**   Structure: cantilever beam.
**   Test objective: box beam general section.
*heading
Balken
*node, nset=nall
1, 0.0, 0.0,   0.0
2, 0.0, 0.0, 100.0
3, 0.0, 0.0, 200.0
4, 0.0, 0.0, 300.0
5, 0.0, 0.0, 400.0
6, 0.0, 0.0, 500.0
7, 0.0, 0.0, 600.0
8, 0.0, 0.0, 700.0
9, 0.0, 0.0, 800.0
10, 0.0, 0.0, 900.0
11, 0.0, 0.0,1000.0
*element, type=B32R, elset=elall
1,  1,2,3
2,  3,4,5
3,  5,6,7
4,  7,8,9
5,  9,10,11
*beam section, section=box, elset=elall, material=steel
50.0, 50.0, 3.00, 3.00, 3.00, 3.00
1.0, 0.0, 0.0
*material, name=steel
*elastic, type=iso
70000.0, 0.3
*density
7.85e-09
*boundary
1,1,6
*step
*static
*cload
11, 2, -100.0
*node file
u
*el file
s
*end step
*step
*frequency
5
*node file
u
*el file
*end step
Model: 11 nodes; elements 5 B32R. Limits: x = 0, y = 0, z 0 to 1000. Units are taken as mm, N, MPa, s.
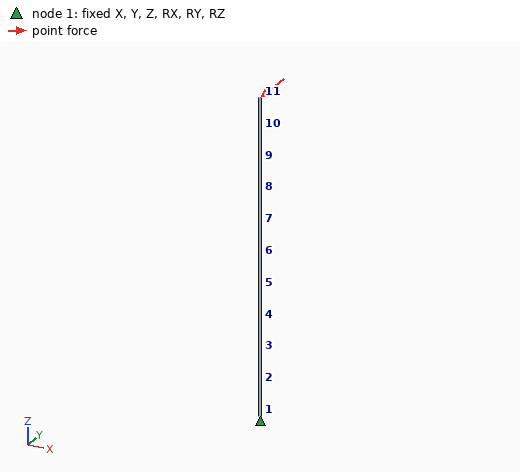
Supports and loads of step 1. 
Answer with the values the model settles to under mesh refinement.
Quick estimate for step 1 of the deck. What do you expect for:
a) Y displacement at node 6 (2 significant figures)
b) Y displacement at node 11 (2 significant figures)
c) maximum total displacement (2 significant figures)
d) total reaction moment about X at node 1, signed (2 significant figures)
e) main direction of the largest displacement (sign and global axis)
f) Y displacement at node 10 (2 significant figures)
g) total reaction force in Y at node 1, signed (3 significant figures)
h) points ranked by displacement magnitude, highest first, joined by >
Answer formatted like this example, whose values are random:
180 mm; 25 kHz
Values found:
-0.72 mm; -2.3 mm; 2.3 mm; -100000 N·mm; -Y; -2.0 mm; 100 N; node 11 > node 10 > node 8 > node 6 > node 1
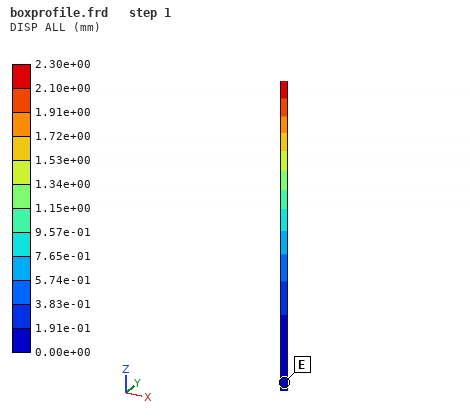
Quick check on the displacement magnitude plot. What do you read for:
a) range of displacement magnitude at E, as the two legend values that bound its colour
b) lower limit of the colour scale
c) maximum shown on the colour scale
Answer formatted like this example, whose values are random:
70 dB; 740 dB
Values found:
0.00e+00 to 1.91e-01 mm; 0.00e+00 mm; 2.30e+00 mm
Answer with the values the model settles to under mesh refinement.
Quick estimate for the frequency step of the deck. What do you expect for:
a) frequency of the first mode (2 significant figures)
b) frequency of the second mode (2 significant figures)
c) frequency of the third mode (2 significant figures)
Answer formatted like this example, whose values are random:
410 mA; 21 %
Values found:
32 Hz; 32 Hz; 190 Hz
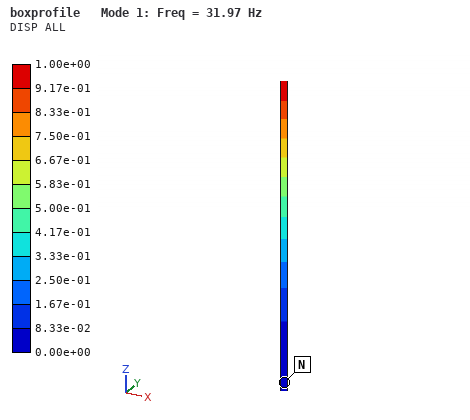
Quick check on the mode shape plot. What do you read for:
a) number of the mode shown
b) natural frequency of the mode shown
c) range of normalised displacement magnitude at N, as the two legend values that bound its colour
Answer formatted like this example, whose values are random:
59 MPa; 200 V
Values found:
1; 31.97 Hz; 0.00e+00 to 8.33e-02
